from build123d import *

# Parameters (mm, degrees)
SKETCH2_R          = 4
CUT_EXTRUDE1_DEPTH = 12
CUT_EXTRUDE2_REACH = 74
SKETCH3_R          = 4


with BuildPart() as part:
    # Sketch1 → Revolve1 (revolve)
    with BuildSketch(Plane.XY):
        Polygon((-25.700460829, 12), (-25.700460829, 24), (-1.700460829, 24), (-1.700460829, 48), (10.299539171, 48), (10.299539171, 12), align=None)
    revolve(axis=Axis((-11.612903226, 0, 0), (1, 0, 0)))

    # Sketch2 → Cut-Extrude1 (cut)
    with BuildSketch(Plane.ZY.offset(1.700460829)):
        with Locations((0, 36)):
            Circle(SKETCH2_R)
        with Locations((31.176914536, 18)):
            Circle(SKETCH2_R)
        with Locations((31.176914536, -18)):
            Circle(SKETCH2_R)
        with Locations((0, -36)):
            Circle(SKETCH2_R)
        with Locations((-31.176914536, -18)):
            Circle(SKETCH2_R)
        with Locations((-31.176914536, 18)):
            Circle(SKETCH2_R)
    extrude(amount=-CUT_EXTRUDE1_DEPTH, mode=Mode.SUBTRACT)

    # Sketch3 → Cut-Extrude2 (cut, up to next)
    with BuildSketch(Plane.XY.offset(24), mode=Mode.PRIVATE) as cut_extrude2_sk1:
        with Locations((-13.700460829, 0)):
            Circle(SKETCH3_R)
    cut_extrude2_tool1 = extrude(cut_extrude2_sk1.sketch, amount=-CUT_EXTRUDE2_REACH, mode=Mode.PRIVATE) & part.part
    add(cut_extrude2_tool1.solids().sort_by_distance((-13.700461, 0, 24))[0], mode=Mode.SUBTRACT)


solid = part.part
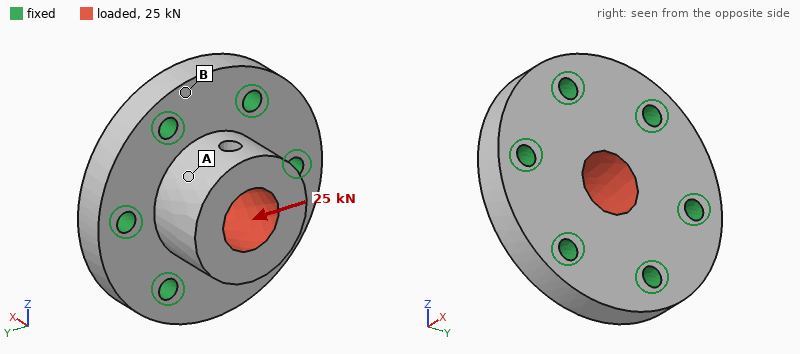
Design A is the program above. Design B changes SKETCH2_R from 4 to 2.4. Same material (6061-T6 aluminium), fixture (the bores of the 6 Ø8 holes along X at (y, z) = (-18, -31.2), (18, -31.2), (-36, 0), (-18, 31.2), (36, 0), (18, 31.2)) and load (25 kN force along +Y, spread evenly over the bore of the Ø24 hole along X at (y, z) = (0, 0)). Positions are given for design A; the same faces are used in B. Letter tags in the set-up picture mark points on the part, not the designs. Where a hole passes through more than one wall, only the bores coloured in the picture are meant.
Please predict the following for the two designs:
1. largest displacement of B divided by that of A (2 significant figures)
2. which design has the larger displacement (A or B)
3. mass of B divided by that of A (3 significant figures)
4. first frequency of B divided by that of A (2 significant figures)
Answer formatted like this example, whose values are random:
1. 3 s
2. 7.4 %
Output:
1. 1.1
2. B
3. 1.02
4. 0.93
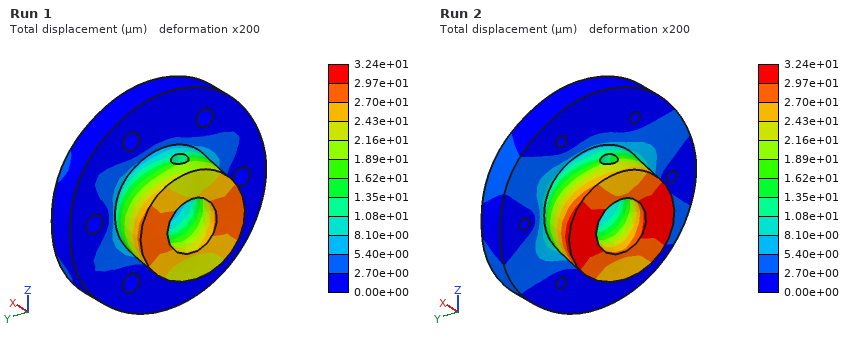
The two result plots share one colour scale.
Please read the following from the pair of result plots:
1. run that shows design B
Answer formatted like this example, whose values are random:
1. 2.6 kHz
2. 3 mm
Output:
1. Run 2
